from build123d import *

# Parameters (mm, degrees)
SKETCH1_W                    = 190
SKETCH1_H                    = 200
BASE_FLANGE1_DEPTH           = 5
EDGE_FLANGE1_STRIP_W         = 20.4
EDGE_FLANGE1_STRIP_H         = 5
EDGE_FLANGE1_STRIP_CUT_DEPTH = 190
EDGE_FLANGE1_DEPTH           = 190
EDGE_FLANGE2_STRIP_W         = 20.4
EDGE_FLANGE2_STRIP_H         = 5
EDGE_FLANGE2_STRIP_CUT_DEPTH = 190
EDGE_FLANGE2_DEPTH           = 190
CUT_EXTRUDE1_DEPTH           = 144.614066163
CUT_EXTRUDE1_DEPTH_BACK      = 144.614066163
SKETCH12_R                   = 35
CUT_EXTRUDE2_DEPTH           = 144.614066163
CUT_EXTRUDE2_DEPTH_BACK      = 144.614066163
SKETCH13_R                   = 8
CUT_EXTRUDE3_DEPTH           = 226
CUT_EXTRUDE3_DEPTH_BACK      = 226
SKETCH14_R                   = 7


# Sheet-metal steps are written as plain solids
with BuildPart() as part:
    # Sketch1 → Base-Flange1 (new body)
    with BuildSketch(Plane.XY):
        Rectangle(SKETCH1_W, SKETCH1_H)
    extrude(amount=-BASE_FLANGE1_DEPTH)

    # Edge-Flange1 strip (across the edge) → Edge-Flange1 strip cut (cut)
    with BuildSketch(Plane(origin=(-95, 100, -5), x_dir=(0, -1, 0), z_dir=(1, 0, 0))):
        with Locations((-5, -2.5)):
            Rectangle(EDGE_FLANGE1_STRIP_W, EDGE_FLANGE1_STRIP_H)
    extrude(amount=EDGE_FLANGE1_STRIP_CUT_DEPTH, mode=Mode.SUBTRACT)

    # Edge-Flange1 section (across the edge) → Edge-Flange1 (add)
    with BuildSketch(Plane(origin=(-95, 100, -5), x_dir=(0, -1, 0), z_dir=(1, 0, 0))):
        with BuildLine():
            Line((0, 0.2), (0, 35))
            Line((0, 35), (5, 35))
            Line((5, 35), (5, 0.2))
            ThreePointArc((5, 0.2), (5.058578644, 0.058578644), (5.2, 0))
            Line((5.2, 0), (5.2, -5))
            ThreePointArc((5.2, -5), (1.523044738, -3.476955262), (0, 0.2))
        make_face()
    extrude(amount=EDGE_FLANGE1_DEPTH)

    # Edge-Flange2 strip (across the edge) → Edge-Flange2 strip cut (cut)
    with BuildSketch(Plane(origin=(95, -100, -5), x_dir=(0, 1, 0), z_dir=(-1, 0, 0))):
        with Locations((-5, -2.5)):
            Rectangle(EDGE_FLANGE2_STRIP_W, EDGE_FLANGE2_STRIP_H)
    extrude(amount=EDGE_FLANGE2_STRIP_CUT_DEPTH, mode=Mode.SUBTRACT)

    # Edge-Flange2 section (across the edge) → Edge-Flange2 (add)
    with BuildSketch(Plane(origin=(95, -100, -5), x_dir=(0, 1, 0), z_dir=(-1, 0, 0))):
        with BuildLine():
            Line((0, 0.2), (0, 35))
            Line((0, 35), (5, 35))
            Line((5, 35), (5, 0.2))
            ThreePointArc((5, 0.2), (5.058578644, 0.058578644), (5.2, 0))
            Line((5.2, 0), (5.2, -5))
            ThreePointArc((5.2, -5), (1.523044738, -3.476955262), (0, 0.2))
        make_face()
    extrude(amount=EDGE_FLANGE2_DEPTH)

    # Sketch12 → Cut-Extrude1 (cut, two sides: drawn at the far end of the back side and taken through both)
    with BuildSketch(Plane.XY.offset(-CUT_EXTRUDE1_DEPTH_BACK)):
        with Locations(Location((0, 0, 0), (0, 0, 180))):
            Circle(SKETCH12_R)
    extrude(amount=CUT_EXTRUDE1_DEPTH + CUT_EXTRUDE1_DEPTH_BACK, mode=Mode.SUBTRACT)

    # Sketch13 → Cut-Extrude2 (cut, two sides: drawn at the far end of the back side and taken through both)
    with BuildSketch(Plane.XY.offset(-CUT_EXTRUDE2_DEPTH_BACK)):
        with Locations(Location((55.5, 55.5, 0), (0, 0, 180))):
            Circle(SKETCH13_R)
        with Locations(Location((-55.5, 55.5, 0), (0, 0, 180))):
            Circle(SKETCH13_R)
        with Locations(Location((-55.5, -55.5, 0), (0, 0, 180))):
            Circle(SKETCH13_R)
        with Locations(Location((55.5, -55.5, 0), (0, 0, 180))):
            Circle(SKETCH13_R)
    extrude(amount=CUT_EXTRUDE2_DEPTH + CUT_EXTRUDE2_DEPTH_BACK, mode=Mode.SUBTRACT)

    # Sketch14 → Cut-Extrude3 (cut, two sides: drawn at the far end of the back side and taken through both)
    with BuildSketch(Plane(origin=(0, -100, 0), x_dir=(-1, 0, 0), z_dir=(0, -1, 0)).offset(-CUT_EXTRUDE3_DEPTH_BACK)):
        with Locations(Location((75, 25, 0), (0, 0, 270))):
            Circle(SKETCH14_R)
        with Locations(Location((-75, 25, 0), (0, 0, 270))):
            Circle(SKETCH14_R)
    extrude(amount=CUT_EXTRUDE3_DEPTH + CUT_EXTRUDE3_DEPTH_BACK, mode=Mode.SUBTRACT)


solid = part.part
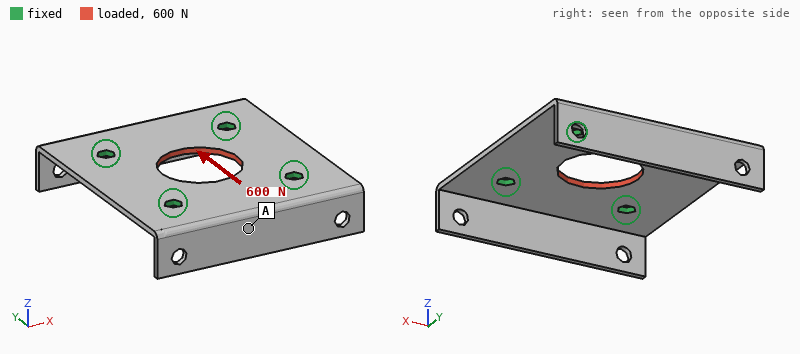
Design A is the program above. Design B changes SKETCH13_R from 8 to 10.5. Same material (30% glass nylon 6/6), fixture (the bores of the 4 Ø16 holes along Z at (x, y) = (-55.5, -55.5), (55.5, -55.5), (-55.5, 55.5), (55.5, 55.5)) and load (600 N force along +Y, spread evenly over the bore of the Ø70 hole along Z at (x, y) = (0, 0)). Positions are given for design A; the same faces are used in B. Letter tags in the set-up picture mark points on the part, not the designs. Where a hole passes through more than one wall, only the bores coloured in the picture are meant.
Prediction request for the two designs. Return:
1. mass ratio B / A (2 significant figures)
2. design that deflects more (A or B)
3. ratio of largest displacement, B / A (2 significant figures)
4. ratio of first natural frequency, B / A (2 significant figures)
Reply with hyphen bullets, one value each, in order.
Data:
- 0.99
- A
- 0.91
- 1.1
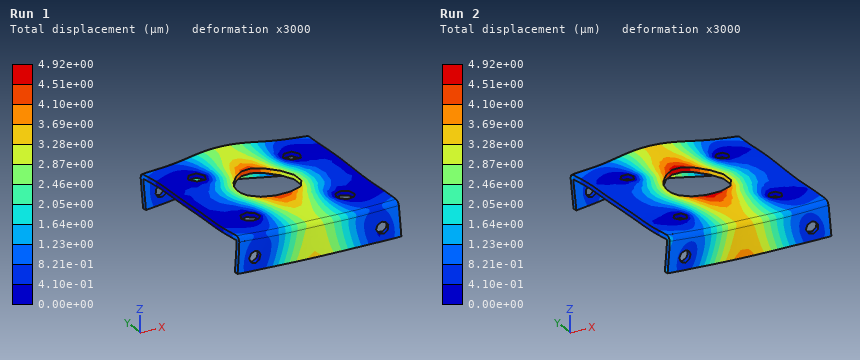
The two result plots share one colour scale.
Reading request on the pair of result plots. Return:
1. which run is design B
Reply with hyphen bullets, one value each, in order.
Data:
- Run 1
